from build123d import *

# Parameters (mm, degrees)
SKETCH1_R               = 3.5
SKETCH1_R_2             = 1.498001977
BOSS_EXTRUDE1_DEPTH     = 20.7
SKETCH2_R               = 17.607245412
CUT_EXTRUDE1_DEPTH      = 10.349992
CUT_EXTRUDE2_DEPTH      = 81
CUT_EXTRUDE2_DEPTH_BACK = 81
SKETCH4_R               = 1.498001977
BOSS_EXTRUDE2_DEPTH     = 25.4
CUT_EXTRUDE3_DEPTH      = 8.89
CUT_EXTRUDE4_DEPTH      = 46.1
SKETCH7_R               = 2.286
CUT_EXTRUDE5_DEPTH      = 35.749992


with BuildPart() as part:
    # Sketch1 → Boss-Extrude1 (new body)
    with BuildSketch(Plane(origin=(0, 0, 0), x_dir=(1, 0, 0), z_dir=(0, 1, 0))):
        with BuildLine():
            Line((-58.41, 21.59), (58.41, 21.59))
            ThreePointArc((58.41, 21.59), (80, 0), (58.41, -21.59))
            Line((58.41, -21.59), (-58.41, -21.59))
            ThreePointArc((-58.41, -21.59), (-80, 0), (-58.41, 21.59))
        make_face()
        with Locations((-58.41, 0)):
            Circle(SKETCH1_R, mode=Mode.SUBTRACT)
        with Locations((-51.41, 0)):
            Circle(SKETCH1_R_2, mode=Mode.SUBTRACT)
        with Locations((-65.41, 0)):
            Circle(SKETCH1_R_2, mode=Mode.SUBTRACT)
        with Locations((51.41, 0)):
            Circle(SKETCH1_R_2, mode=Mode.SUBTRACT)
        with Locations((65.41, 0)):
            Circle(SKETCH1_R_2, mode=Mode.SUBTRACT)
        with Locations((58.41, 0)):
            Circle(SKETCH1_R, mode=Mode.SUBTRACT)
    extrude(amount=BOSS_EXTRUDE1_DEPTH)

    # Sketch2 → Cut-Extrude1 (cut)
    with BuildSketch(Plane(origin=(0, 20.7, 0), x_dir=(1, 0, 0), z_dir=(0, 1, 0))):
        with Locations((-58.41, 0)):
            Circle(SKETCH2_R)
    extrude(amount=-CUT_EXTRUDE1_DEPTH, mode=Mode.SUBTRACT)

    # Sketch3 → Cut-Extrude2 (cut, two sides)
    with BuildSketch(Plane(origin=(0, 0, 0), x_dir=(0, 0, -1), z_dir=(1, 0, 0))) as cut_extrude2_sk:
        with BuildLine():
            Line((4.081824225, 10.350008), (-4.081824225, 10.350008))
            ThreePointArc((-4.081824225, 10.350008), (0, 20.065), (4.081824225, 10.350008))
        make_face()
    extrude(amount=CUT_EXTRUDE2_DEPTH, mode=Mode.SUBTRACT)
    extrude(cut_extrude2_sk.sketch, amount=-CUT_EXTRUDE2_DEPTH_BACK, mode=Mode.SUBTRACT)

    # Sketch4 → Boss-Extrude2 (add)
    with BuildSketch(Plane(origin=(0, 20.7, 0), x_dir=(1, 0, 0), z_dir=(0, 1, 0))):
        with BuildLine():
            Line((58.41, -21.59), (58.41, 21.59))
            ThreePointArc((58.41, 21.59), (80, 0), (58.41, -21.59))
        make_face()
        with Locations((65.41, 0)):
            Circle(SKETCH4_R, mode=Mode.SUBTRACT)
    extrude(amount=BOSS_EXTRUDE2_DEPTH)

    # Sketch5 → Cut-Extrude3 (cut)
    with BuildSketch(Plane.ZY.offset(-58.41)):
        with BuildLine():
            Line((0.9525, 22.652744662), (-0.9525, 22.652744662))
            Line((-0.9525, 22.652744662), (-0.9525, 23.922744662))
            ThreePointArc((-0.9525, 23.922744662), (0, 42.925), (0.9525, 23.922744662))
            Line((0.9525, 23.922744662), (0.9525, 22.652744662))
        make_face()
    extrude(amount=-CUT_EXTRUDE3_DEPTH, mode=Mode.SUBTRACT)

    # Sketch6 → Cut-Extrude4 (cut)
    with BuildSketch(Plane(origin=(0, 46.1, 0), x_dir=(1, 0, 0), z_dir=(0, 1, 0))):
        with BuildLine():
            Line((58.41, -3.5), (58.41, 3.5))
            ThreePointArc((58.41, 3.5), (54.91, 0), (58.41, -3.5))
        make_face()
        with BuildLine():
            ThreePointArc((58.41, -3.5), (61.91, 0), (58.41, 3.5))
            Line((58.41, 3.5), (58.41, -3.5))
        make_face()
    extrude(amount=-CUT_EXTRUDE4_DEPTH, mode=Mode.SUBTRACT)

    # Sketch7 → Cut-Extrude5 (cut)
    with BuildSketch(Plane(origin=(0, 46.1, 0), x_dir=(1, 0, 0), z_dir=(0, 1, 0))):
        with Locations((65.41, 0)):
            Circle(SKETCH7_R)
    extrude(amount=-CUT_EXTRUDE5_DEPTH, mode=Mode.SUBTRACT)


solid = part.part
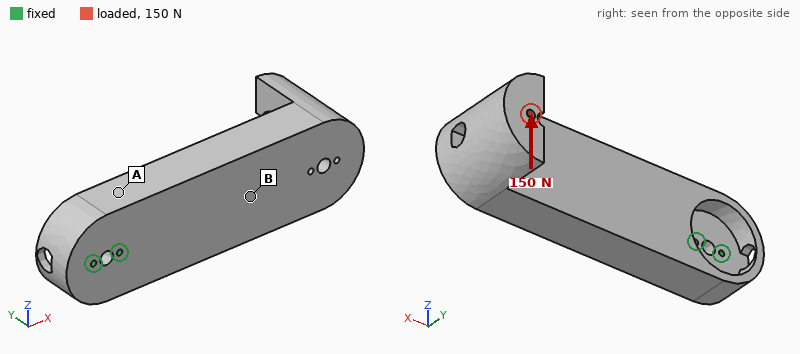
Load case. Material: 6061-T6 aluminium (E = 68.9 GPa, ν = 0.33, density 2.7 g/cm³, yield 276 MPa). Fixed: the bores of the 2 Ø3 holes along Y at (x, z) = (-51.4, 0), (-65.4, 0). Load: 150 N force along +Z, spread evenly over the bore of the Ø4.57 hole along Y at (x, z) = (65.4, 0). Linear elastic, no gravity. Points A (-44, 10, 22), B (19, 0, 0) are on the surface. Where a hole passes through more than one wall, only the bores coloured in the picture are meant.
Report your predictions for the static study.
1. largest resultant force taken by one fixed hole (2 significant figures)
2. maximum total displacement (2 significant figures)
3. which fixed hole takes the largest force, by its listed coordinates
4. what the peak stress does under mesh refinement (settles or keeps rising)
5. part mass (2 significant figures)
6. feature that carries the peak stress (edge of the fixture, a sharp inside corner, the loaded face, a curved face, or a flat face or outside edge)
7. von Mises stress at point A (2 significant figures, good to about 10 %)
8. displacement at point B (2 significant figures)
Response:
1.2 kN
54 µm
(-51.4, 0)
keeps rising
340 g
edge of the fixture
3.9 MPa
18 µm
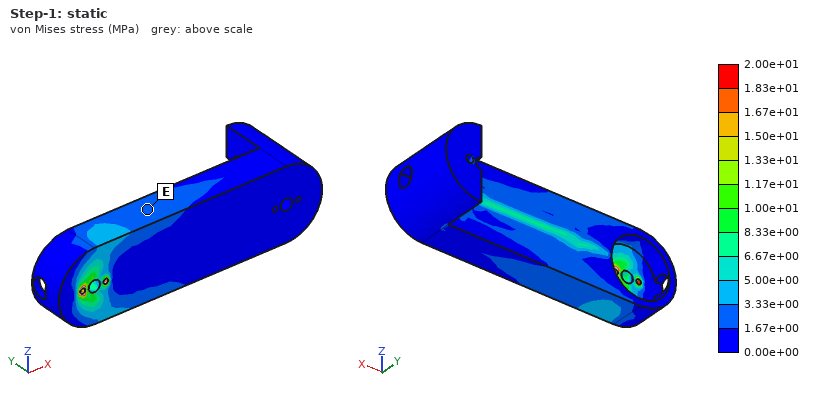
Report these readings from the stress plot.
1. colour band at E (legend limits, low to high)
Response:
1.67e+00 to 3.33e+00 MPa
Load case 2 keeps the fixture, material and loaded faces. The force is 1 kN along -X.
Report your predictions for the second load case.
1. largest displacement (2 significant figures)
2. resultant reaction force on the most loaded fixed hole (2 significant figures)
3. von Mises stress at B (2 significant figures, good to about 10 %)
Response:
0.22 mm
1.2 kN
6.3 MPa
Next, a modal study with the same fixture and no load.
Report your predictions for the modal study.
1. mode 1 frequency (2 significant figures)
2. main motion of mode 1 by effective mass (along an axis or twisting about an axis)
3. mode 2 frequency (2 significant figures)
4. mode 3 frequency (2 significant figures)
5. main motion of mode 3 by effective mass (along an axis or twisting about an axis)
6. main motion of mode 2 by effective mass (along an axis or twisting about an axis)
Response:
520 Hz
along Y
830 Hz
2100 Hz
twisting about X
along Z
